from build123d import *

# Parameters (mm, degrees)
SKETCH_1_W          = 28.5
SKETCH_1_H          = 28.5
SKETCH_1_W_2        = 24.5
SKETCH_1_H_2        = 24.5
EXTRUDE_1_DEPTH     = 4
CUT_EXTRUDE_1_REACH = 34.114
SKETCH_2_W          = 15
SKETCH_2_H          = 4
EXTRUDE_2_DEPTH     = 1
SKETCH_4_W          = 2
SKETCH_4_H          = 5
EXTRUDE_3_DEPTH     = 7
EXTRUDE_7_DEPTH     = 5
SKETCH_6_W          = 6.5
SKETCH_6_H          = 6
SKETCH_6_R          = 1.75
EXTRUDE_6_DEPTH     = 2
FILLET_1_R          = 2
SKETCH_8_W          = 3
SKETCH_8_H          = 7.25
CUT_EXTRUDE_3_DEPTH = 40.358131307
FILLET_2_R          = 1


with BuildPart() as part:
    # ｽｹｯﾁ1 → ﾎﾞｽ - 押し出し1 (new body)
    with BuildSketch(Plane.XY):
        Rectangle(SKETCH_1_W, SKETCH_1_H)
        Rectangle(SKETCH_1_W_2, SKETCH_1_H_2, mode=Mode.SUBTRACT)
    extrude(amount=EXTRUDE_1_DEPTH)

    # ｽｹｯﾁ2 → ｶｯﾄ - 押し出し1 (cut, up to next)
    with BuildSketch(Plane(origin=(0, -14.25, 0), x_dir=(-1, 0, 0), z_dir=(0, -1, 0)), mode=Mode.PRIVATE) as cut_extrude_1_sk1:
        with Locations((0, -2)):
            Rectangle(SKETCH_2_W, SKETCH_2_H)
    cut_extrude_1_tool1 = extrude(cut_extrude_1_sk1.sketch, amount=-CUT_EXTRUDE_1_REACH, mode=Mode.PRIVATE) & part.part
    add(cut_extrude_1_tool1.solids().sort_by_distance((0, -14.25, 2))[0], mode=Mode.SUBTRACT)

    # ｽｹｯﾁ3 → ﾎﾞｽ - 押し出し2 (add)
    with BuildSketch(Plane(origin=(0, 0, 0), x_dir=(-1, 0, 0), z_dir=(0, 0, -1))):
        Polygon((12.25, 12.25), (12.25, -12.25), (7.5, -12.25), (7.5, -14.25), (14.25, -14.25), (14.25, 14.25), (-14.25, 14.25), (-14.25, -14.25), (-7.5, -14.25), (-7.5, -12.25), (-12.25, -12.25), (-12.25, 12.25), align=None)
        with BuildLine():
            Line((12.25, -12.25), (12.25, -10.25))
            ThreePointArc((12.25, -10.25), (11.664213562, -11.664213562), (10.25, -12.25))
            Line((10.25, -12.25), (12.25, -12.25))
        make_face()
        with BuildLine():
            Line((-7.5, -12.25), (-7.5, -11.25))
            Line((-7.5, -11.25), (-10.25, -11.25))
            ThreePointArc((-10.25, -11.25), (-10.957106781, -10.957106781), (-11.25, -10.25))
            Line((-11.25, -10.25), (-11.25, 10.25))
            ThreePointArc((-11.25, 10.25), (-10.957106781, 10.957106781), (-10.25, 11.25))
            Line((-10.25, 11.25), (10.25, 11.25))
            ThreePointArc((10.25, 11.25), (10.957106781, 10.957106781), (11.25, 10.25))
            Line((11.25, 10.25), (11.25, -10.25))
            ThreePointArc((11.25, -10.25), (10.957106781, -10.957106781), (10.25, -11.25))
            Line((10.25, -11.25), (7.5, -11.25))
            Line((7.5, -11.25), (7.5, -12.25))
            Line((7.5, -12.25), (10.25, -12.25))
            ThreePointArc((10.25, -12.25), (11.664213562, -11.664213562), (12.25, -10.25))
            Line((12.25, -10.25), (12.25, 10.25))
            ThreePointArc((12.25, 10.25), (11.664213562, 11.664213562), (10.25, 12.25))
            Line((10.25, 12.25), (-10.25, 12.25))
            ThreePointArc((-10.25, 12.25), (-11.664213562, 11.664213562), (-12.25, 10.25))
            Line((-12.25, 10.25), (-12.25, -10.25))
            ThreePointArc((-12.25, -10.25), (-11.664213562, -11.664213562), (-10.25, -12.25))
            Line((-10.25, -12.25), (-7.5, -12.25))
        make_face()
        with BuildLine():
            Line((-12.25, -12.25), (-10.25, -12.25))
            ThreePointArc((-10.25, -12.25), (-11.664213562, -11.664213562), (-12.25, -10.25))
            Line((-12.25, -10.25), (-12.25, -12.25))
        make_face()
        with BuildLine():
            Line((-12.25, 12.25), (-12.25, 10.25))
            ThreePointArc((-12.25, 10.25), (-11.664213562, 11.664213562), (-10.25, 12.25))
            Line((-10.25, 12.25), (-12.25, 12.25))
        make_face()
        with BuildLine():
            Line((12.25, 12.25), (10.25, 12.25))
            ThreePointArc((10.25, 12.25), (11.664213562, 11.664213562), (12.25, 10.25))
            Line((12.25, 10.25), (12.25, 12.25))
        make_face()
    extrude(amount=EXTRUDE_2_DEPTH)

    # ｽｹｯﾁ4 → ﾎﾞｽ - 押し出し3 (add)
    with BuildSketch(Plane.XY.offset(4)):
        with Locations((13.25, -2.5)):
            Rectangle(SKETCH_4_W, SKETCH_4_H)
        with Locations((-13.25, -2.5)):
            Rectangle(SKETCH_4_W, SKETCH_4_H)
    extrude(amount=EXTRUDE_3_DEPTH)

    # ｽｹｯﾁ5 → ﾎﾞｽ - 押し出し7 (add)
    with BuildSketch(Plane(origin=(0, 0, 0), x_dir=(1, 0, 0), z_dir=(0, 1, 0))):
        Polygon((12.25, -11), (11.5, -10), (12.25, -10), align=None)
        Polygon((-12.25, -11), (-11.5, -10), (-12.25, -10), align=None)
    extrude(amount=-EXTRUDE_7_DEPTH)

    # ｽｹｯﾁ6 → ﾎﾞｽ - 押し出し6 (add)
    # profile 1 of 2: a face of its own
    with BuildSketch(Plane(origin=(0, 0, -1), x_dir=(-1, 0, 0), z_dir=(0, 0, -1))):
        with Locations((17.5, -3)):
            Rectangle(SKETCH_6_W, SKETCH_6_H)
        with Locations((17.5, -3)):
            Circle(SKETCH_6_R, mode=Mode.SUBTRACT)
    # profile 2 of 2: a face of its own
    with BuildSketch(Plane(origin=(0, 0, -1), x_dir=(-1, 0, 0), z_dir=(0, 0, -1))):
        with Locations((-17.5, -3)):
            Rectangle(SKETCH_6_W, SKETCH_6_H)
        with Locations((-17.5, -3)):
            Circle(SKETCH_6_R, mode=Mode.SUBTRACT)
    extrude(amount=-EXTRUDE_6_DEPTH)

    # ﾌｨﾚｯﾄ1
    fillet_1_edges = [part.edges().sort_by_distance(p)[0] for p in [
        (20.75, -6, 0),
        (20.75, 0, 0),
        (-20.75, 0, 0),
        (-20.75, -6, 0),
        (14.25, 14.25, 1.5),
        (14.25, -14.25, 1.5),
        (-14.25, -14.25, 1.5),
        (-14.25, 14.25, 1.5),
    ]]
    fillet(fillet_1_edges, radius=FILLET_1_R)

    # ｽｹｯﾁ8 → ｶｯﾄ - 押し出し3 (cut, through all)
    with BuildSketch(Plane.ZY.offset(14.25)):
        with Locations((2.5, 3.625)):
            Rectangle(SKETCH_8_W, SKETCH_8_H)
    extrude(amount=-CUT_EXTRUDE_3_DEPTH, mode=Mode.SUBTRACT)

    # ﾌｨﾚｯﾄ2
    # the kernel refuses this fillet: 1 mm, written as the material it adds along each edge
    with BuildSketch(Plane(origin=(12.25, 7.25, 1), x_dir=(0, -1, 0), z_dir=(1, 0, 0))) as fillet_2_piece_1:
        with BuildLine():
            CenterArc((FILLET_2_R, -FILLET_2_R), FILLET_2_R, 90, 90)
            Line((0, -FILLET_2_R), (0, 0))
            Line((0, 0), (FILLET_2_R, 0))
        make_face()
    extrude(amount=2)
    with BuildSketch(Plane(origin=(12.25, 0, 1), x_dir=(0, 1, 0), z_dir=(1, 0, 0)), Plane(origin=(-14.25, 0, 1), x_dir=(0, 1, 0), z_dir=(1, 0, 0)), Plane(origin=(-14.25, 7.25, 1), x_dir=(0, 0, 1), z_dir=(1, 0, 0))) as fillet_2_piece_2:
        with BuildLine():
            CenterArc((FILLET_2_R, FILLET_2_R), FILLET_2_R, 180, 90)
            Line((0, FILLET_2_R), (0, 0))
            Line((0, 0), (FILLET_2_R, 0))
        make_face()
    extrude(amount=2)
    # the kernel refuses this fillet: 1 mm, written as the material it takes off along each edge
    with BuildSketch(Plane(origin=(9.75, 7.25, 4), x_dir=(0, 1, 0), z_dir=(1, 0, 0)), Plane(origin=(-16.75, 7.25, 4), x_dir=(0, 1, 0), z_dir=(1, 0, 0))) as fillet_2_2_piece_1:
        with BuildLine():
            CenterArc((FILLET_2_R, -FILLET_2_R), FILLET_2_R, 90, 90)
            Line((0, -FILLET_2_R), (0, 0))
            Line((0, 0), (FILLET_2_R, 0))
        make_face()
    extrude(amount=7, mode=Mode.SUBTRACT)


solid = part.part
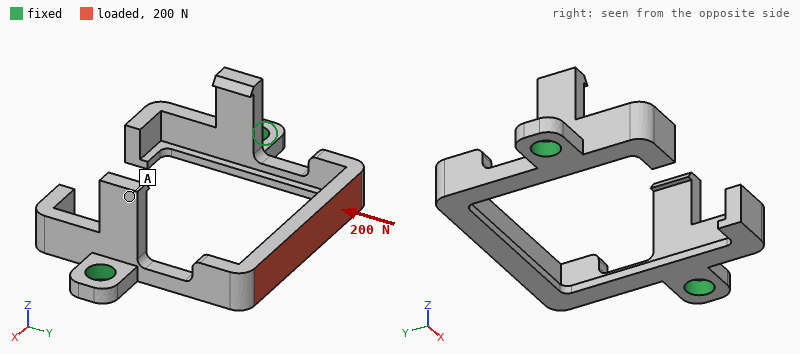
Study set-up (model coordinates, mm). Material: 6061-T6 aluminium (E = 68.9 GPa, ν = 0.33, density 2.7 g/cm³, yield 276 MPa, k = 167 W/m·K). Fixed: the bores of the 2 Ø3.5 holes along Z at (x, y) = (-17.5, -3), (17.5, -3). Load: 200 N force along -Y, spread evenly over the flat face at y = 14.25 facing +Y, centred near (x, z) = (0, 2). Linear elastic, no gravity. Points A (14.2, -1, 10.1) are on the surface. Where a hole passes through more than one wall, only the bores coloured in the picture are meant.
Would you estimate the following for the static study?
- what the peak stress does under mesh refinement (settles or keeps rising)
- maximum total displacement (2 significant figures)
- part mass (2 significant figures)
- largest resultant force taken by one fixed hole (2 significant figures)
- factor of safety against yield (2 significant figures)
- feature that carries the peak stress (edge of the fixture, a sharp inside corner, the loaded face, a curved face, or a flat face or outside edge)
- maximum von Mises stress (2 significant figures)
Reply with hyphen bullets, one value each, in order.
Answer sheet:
- settles
- 0.19 mm
- 3.1 g
- 110 N
- 1.2
- a curved face
- 230 MPa
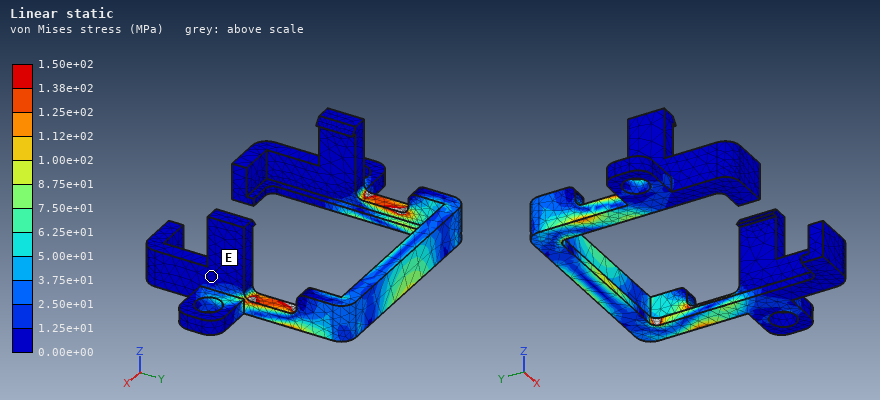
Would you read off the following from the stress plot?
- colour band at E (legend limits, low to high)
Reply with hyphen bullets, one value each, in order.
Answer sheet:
- 0.00e+00 to 1.25e+01 MPa
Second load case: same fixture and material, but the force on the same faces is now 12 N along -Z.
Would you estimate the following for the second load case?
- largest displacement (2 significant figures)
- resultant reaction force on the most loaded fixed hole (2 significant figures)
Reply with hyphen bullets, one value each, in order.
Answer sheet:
- 71 µm
- 6.2 N
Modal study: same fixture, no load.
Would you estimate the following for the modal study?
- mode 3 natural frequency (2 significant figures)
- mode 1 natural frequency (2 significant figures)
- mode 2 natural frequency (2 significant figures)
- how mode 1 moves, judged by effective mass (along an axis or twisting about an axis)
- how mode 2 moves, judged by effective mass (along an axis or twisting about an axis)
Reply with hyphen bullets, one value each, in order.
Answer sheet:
- 6200 Hz
- 2400 Hz
- 5100 Hz
- along Z
- along X
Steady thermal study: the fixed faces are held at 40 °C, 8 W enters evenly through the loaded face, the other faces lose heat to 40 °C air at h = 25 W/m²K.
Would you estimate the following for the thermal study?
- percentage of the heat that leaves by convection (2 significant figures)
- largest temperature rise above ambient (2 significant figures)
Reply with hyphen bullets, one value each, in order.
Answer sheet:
- 11 %
- 67 K
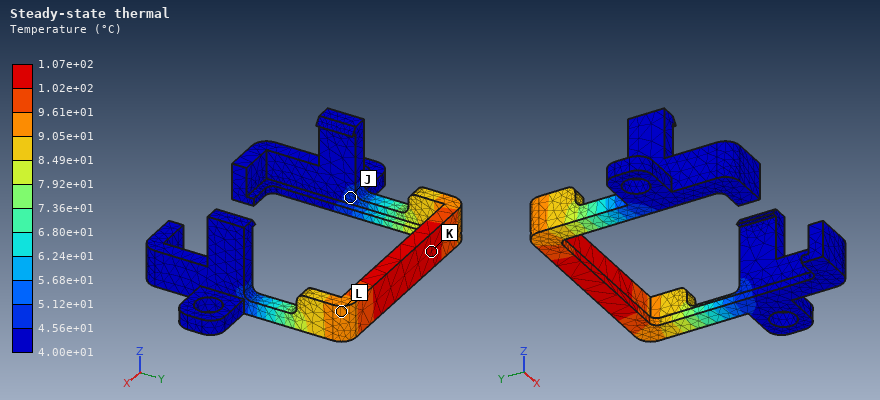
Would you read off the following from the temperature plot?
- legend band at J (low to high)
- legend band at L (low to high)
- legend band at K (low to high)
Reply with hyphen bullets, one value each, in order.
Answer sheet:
- 4.56e+01 to 5.12e+01 °C
- 9.05e+01 to 9.61e+01 °C
- 1.02e+02 to 1.07e+02 °C
